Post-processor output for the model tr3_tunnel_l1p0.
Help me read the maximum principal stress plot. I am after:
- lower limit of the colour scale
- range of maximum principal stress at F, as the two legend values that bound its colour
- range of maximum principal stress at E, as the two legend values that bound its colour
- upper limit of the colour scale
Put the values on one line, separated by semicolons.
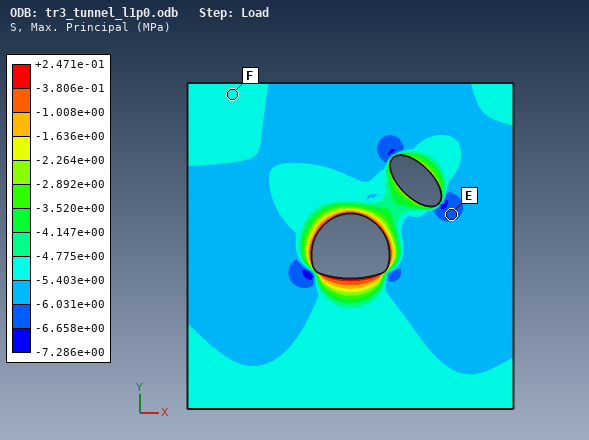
-7.286e+00 MPa; -5.403e+00 to -4.775e+00 MPa; -6.658e+00 to -6.031e+00 MPa; +2.471e-01 MPa
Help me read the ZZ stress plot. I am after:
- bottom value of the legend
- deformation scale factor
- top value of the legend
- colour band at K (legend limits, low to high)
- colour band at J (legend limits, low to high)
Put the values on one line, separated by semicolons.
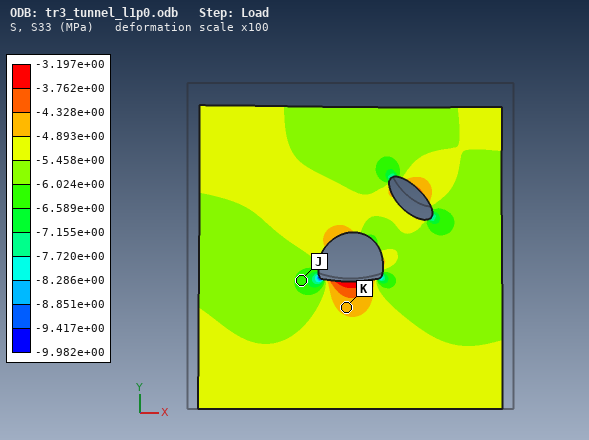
-9.982e+00 MPa; 100; -3.197e+00 MPa; -4.893e+00 to -4.328e+00 MPa; -6.589e+00 to -6.024e+00 MPa
